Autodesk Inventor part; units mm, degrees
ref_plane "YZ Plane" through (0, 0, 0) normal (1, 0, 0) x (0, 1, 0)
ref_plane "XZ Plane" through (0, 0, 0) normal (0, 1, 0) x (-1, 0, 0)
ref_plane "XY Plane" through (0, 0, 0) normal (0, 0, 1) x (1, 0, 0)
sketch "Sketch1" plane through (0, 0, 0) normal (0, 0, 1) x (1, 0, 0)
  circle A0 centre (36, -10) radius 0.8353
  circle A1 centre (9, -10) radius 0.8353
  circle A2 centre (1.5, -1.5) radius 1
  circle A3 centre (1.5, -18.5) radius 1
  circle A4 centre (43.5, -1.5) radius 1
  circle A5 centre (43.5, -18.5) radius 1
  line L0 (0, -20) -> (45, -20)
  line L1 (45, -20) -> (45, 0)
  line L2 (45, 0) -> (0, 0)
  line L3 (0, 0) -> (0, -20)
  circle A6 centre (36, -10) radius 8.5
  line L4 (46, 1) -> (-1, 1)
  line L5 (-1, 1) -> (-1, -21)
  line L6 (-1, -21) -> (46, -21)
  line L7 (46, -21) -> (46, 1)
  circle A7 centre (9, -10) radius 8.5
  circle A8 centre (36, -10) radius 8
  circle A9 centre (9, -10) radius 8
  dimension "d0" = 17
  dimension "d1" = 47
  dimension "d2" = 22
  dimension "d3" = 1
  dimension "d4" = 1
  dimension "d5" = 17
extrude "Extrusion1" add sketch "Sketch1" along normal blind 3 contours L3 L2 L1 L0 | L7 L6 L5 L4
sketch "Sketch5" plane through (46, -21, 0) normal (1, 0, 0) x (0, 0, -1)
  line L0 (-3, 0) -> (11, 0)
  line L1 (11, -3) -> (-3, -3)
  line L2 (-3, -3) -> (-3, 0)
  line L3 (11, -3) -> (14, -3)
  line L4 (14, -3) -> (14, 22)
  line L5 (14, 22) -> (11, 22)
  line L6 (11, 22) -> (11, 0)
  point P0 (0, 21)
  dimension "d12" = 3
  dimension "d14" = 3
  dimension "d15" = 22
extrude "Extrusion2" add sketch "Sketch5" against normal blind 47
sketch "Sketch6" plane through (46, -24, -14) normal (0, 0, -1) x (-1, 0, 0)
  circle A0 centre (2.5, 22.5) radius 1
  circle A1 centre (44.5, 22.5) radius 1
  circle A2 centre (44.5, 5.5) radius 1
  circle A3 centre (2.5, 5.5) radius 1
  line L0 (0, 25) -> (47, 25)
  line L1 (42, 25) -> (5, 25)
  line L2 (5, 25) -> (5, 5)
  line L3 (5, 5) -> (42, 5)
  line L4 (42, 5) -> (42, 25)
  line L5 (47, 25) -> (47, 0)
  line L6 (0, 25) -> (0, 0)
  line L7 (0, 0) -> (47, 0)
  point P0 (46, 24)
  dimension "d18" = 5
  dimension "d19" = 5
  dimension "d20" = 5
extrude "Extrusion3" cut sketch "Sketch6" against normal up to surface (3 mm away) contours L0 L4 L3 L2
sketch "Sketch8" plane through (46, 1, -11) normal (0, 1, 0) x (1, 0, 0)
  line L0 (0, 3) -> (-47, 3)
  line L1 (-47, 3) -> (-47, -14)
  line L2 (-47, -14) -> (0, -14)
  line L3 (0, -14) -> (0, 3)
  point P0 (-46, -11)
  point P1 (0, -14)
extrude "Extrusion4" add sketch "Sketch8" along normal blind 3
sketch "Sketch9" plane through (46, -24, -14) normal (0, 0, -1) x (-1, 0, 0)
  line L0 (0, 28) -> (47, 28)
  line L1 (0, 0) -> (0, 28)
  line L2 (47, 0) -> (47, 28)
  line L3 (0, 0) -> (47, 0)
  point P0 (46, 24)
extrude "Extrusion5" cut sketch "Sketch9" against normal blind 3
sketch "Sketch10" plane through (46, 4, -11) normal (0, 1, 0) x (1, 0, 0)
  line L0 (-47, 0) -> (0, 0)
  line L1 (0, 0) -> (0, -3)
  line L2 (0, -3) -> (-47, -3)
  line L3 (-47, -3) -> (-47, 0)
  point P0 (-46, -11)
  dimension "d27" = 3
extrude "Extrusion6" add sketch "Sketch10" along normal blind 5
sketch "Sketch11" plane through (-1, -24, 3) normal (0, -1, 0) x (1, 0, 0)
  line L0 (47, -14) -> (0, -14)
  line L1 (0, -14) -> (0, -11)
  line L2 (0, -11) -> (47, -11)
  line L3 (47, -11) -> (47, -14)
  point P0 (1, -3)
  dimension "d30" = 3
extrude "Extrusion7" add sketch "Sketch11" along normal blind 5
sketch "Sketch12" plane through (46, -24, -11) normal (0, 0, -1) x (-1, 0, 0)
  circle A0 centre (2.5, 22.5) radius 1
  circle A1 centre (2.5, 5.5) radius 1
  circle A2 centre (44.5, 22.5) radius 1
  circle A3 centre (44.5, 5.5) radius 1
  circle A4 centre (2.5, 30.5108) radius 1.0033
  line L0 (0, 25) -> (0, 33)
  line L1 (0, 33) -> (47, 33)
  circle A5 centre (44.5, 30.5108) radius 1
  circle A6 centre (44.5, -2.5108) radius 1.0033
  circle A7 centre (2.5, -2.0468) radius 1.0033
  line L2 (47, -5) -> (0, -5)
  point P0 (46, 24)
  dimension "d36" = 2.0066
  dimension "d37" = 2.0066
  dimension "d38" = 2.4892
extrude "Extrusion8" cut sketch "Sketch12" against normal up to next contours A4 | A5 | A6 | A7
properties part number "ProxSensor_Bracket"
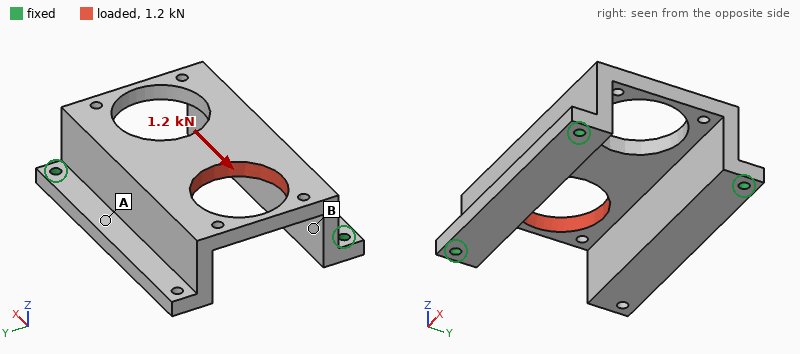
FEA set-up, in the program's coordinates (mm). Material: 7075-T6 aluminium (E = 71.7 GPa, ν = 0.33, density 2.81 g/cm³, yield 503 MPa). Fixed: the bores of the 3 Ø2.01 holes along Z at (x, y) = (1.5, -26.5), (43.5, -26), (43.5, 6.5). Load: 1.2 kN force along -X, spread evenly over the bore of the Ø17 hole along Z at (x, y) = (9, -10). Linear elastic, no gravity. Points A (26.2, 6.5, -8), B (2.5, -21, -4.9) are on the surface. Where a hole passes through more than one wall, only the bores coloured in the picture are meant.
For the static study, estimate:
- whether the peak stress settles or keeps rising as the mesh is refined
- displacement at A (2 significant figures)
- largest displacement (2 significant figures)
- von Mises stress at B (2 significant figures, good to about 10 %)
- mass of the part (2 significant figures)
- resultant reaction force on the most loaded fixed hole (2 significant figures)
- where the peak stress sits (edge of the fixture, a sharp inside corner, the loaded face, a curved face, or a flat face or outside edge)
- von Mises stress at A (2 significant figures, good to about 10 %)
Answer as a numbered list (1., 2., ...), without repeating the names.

1. keeps rising
2. 0.044 mm
3. 0.13 mm
4. 24 MPa
5. 20 g
6. 550 N
7. edge of the fixture
8. 9.8 MPa
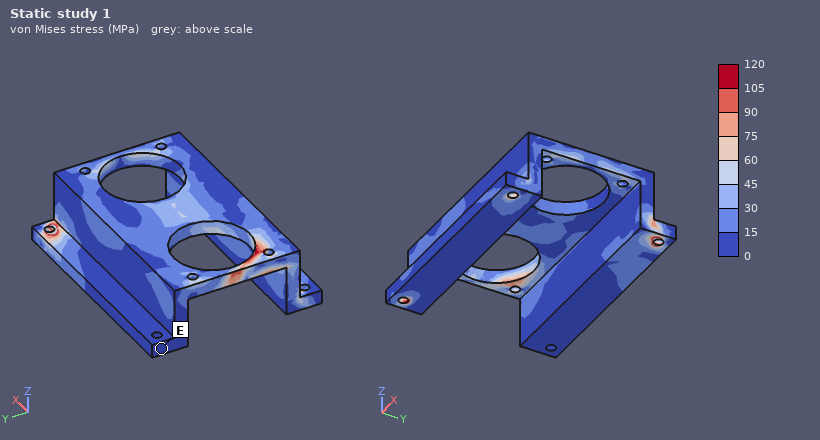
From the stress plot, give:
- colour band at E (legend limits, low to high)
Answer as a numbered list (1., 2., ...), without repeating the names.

1. 0 to 15 MPa
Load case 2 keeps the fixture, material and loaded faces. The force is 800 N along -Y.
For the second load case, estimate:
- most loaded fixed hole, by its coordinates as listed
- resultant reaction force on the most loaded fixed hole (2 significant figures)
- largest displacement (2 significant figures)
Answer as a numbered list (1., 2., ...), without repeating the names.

1. (43.5, 6.5)
2. 560 N
3. 99 µm
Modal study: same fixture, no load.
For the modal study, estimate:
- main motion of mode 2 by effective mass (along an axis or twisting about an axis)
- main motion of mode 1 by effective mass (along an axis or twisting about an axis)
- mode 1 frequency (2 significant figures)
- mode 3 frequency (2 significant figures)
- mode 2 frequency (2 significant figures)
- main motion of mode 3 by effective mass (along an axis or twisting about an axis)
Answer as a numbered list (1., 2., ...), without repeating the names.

1. along Y
2. along Z
3. 2800 Hz
4. 8600 Hz
5. 5000 Hz
6. along Y
